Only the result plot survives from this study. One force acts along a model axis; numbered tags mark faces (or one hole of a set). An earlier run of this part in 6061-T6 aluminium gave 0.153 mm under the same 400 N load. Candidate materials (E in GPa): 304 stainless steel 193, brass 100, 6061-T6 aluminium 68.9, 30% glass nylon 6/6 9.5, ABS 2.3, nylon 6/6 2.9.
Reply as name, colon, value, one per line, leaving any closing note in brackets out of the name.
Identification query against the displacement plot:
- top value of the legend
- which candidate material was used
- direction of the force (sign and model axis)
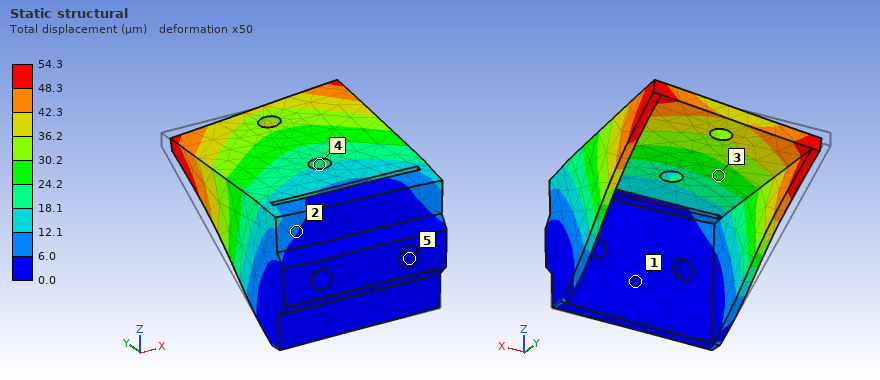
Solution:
top value of the legend: 54.3 µm
which candidate material was used: 304 stainless steel
direction of the force: +X
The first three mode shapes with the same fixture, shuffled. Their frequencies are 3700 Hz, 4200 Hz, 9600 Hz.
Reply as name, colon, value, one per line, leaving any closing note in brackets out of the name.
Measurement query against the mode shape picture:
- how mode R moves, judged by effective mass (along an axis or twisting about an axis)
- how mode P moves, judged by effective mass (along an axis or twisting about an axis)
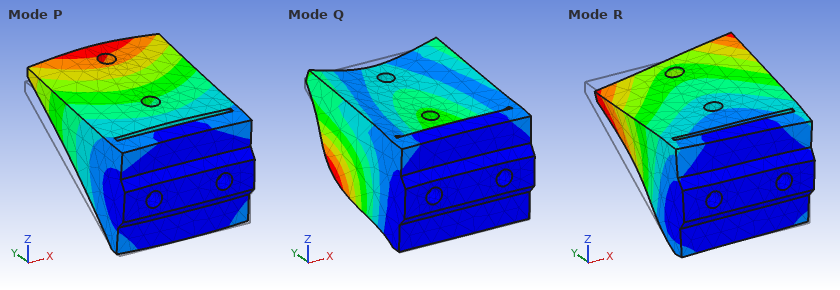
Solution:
how mode R moves, judged by effective mass: along X
how mode P moves, judged by effective mass: along Z
